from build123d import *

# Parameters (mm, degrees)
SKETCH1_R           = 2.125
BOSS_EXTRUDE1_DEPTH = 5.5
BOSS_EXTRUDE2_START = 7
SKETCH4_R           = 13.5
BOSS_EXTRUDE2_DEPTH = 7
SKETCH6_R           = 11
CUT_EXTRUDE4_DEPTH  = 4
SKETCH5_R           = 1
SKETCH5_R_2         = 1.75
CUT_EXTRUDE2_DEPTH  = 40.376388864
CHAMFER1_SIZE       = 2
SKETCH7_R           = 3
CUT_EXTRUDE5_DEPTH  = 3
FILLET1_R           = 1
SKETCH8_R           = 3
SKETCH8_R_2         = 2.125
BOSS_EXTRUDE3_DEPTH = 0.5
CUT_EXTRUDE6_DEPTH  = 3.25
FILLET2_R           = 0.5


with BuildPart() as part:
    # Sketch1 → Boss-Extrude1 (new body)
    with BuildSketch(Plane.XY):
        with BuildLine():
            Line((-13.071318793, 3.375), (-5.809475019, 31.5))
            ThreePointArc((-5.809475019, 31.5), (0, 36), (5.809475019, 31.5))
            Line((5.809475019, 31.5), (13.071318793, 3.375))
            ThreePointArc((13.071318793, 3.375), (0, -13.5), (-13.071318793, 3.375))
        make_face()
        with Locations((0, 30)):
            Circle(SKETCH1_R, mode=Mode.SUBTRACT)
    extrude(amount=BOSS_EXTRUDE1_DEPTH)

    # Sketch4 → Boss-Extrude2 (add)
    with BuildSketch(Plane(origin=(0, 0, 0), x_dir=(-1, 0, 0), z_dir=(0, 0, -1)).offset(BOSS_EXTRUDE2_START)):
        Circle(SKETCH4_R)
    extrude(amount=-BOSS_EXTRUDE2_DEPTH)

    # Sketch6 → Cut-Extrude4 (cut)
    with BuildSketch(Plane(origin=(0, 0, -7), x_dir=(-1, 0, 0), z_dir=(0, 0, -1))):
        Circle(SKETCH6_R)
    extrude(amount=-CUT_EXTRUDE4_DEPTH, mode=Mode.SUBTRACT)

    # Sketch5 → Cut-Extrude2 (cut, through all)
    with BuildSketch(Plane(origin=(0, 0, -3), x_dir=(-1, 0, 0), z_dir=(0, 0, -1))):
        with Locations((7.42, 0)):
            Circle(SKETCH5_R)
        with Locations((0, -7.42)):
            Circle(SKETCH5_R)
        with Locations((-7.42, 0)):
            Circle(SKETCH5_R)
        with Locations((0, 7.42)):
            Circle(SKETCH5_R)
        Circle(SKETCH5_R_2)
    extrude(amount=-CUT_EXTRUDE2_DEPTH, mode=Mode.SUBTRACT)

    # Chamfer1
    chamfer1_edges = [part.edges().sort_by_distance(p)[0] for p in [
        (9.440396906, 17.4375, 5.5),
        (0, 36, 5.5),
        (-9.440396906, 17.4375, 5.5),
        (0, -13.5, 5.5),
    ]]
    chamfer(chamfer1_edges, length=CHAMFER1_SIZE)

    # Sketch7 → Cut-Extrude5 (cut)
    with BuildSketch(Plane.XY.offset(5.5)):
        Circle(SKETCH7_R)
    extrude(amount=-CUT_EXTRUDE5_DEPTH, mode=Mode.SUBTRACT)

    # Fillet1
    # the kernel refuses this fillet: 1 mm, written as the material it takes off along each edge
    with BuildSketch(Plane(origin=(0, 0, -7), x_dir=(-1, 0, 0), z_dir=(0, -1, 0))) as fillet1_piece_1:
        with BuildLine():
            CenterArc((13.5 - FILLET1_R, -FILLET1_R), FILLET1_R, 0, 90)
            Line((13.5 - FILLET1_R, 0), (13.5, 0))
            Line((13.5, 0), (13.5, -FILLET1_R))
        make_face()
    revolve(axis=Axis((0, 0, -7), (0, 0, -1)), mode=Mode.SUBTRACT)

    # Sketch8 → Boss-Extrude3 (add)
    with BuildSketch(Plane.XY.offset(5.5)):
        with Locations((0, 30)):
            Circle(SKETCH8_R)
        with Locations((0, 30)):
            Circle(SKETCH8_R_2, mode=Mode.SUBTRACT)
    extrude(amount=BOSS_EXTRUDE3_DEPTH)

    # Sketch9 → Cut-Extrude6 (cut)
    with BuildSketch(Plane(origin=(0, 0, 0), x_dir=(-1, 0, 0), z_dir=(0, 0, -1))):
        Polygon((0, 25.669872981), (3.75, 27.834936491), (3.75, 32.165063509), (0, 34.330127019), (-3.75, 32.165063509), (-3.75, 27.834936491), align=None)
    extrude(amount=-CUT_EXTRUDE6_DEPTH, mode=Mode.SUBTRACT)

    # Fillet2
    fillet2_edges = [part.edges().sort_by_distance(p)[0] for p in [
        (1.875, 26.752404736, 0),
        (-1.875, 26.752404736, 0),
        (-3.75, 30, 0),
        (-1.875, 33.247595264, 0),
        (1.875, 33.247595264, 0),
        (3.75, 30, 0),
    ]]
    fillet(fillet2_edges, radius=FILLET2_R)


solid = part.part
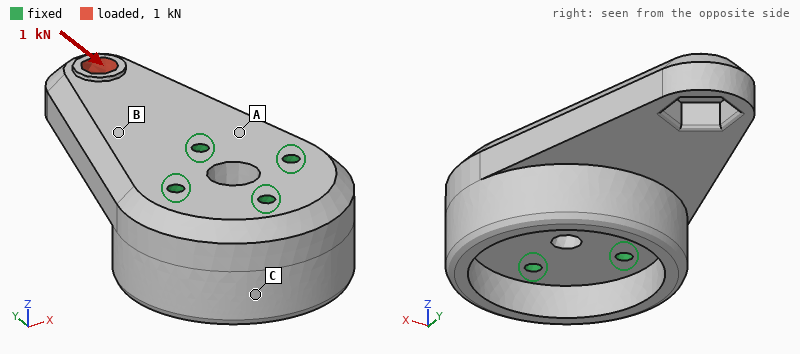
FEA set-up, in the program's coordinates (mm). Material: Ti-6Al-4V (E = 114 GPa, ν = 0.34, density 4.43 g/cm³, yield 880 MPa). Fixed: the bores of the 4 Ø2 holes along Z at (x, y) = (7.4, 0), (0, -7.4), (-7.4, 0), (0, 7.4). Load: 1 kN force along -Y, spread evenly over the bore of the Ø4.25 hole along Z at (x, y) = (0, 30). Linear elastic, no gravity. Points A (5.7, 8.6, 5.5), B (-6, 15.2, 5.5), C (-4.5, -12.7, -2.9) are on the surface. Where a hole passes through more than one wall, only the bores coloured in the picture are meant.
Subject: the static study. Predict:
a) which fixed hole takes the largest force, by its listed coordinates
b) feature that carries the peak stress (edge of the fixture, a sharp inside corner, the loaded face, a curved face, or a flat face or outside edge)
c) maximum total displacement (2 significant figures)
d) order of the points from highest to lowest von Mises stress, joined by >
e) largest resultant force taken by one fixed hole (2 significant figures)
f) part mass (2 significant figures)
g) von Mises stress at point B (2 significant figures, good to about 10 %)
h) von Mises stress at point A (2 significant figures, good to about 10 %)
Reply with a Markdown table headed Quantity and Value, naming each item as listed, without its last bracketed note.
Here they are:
| Quantity | Value |
|---|---|
| which fixed hole takes the largest force, by its listed coordinates | (0, 7.4) |
| feature that carries the peak stress | the loaded face |
| maximum total displacement | 28 µm |
| order of the points from highest to lowest von Mises stress, joined by > | B > A > C |
| largest resultant force taken by one fixed hole | 540 N |
| part mass | 31 g |
| von Mises stress at point B | 29 MPa |
| von Mises stress at point A | 16 MPa |
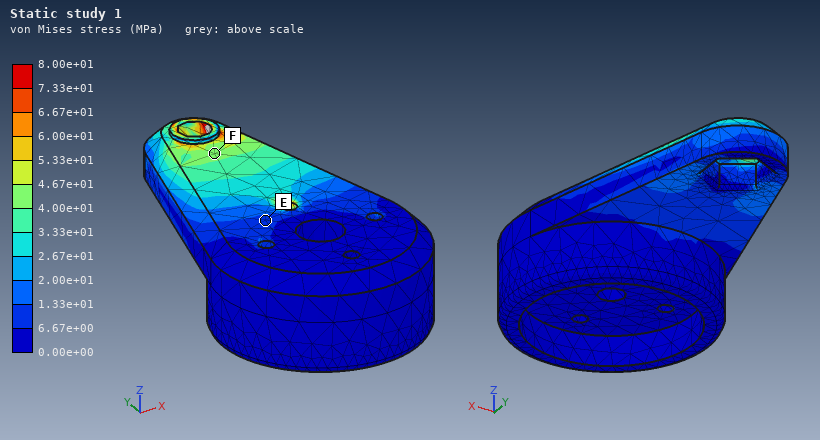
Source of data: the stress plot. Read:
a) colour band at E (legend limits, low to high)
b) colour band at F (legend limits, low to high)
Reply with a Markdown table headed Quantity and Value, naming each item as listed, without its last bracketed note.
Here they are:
| Quantity | Value |
|---|---|
| colour band at E | 6.67e+00 to 1.33e+01 MPa |
| colour band at F | 4.00e+01 to 4.67e+01 MPa |
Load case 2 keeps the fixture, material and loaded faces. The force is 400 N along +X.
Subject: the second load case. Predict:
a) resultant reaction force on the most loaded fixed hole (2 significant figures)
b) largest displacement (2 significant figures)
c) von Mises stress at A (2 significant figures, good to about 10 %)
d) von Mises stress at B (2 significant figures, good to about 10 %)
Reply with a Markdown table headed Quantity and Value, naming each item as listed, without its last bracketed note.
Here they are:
| Quantity | Value |
|---|---|
| resultant reaction force on the most loaded fixed hole | 470 N |
| largest displacement | 11 µm |
| von Mises stress at A | 8.5 MPa |
| von Mises stress at B | 13 MPa |
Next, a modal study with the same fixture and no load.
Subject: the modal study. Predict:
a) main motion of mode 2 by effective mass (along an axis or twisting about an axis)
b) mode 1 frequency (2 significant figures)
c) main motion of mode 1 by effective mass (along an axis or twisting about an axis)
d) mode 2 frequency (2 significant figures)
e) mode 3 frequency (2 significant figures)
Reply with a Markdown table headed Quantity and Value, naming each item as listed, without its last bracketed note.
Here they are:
| Quantity | Value |
|---|---|
| main motion of mode 2 by effective mass | along X |
| mode 1 frequency | 9500 Hz |
| main motion of mode 1 by effective mass | along Z |
| mode 2 frequency | 20 kHz |
| mode 3 frequency | 26 kHz |
